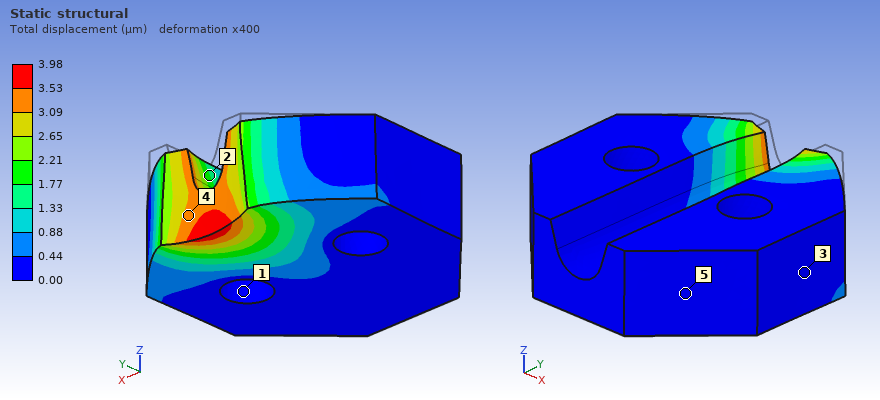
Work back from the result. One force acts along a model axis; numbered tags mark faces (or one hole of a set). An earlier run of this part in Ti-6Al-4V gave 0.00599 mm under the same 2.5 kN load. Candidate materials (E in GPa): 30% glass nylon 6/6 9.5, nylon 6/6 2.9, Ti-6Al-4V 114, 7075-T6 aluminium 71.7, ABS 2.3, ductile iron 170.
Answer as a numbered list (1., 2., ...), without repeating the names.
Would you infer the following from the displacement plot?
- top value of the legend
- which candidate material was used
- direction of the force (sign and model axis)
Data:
1. 3.98 µm
2. ductile iron
3. -Y
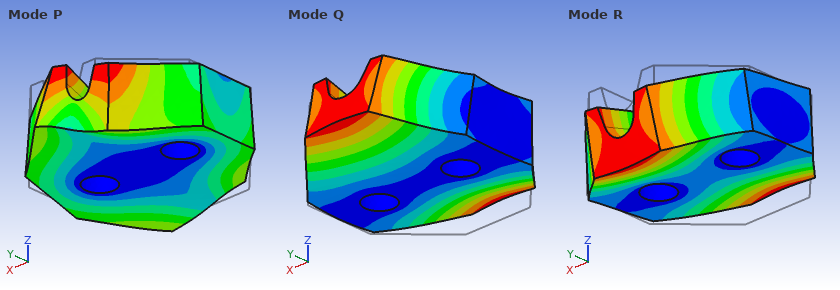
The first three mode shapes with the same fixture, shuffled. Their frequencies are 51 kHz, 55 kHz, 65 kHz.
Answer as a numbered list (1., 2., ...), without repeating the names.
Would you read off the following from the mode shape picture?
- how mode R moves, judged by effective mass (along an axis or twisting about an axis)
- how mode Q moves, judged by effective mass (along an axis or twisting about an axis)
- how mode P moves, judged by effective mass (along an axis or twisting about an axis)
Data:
1. twisting about X
2. along Z
3. twisting about Z
